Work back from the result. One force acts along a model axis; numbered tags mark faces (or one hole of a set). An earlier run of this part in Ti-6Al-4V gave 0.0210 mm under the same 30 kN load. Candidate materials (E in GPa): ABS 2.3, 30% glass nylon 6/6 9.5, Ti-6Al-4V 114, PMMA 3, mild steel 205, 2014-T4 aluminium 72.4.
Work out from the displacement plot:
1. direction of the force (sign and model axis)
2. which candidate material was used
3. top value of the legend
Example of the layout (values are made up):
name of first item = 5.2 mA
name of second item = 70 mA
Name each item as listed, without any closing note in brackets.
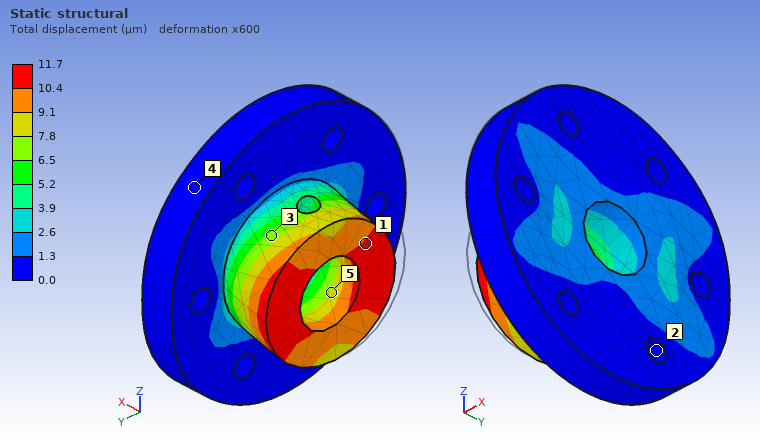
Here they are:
direction of the force = +Y
which candidate material was used = mild steel
top value of the legend = 11.7 µm
